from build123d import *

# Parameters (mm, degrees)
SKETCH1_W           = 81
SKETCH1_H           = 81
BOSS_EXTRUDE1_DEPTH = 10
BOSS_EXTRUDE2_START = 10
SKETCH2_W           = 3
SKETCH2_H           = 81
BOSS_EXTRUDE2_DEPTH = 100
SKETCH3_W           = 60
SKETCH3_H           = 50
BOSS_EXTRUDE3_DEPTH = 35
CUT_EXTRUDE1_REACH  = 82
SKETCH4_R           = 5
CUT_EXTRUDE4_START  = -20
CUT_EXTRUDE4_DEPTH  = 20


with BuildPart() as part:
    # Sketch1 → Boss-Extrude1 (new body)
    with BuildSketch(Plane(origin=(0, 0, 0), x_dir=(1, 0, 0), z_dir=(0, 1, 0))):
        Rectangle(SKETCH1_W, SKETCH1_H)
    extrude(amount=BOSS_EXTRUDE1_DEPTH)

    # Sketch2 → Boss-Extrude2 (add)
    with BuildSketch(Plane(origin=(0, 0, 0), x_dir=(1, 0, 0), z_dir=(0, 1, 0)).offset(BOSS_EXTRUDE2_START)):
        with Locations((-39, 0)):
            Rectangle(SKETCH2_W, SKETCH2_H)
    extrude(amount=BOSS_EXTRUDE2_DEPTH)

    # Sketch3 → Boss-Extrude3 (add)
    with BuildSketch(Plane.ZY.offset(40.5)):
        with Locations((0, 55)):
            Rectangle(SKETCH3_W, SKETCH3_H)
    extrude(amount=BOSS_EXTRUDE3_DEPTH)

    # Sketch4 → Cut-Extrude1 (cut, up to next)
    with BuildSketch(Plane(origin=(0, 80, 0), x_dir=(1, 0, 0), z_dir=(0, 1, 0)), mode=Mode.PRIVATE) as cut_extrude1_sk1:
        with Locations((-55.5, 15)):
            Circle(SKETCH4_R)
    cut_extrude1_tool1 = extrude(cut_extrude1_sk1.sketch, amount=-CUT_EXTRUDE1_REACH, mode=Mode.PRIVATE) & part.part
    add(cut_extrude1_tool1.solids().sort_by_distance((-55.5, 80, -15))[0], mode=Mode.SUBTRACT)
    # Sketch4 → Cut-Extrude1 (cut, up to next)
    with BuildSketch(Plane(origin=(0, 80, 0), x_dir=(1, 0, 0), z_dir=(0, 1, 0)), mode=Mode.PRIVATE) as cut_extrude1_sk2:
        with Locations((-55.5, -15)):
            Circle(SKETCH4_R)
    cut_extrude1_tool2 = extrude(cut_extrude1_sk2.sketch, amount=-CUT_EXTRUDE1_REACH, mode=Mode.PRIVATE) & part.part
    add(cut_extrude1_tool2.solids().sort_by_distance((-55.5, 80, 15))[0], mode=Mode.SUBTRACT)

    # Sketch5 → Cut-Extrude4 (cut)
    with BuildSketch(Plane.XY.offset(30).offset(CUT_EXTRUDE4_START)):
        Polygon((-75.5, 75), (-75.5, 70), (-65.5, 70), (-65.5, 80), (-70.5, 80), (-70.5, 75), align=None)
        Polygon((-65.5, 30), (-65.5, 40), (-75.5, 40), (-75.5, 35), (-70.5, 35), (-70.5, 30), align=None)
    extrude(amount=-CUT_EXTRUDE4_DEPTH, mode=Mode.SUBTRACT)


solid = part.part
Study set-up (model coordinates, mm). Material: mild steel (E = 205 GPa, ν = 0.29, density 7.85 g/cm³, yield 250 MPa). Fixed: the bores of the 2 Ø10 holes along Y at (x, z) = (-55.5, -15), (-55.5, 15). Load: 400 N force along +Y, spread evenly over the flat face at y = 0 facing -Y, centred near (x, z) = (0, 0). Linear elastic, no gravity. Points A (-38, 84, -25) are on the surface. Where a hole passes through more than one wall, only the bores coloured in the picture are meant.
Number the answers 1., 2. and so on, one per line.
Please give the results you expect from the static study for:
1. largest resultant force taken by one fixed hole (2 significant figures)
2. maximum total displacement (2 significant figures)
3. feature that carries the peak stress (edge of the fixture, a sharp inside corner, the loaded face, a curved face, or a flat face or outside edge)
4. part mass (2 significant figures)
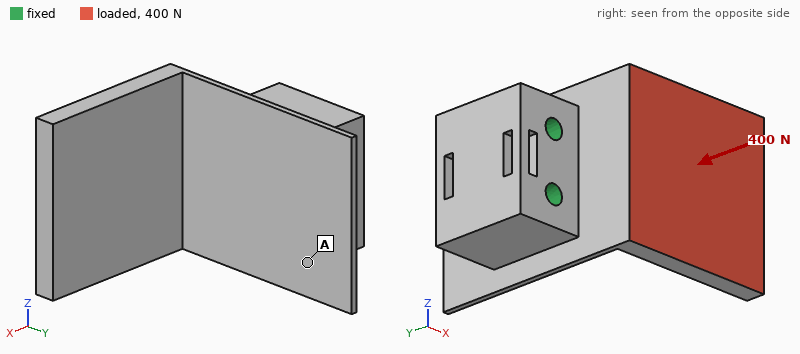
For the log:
1. 200 N
2. 0.72 mm
3. a flat face or outside edge
4. 1.4 kg
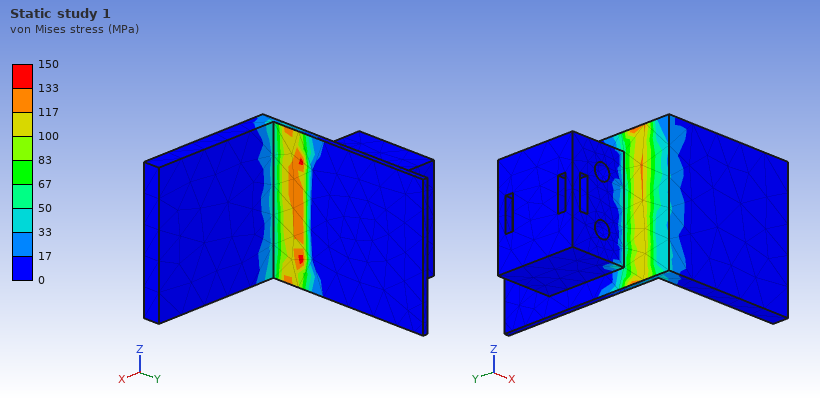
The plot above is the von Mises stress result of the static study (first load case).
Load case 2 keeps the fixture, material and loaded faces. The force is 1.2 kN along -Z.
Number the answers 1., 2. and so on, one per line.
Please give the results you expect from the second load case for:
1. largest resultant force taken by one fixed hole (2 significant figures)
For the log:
1. 2.1 kN
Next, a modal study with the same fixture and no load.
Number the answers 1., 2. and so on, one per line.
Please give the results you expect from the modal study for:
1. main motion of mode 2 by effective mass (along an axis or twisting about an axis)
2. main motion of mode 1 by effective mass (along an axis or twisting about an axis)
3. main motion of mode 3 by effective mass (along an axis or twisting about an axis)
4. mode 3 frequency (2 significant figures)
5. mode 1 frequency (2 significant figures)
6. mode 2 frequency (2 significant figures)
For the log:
1. along Z
2. along Y
3. along X
4. 1400 Hz
5. 190 Hz
6. 610 Hz
